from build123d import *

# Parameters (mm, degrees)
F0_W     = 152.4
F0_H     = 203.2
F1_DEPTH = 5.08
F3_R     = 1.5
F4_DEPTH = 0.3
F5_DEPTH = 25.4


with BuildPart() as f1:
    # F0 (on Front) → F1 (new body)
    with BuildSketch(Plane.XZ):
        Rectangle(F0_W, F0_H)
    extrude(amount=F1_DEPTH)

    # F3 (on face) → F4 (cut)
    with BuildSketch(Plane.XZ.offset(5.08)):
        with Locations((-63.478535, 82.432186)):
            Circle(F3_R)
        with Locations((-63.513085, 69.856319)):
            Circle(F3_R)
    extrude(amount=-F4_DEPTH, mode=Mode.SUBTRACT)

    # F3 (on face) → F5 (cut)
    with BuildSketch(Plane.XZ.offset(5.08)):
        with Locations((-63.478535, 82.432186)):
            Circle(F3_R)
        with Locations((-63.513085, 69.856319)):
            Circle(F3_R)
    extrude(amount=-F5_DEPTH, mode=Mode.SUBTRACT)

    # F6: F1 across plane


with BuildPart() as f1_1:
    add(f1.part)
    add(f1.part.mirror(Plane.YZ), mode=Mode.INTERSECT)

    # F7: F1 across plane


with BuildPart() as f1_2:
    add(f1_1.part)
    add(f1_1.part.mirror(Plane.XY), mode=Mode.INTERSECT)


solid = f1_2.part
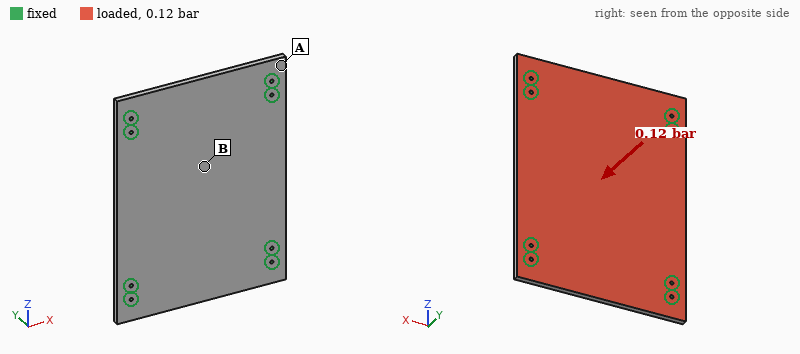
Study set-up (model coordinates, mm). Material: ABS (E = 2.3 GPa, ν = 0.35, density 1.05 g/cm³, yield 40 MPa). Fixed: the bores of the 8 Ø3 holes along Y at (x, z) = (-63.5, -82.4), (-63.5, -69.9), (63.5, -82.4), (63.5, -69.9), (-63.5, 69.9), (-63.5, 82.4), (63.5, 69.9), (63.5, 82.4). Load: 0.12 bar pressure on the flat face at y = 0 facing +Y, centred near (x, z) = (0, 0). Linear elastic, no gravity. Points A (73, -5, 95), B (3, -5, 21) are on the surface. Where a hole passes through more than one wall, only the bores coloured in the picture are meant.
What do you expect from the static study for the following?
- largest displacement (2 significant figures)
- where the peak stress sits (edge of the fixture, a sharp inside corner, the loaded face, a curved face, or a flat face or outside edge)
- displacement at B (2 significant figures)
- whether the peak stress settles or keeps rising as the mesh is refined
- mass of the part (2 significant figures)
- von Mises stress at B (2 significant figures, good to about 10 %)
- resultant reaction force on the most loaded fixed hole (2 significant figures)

1.1 mm
edge of the fixture
1.0 mm
keeps rising
160 g
2.6 MPa
110 N
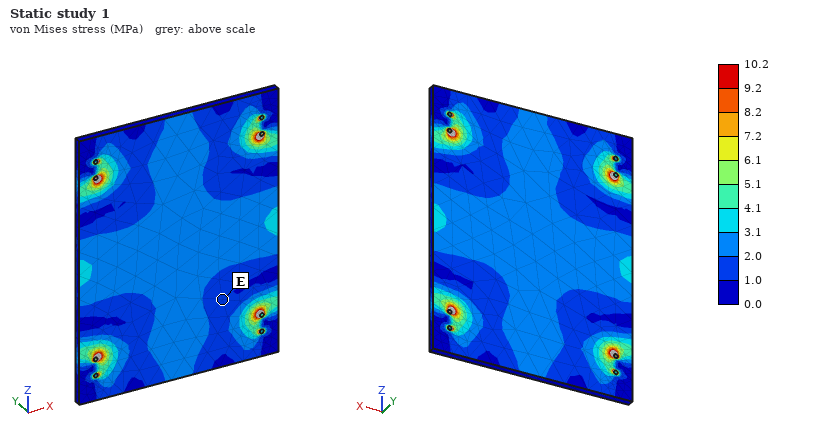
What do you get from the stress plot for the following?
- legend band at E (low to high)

1.0 to 2.0 MPa
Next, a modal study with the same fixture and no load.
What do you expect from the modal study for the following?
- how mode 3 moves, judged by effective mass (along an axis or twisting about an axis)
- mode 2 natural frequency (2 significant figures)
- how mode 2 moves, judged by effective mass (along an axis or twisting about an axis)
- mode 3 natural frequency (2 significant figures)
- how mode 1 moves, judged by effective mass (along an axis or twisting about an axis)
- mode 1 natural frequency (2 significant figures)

twisting about X
430 Hz
twisting about Z
460 Hz
along Y
270 Hz
